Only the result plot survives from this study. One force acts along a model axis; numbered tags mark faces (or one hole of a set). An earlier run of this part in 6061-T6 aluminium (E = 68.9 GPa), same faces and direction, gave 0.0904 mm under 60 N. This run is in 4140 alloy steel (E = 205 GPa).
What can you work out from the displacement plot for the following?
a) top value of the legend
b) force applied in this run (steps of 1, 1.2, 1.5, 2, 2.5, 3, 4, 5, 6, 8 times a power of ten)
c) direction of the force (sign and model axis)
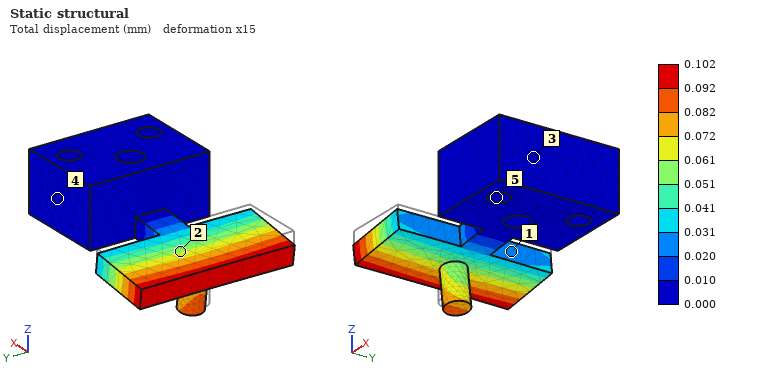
0.102 mm
200 N
-Z
